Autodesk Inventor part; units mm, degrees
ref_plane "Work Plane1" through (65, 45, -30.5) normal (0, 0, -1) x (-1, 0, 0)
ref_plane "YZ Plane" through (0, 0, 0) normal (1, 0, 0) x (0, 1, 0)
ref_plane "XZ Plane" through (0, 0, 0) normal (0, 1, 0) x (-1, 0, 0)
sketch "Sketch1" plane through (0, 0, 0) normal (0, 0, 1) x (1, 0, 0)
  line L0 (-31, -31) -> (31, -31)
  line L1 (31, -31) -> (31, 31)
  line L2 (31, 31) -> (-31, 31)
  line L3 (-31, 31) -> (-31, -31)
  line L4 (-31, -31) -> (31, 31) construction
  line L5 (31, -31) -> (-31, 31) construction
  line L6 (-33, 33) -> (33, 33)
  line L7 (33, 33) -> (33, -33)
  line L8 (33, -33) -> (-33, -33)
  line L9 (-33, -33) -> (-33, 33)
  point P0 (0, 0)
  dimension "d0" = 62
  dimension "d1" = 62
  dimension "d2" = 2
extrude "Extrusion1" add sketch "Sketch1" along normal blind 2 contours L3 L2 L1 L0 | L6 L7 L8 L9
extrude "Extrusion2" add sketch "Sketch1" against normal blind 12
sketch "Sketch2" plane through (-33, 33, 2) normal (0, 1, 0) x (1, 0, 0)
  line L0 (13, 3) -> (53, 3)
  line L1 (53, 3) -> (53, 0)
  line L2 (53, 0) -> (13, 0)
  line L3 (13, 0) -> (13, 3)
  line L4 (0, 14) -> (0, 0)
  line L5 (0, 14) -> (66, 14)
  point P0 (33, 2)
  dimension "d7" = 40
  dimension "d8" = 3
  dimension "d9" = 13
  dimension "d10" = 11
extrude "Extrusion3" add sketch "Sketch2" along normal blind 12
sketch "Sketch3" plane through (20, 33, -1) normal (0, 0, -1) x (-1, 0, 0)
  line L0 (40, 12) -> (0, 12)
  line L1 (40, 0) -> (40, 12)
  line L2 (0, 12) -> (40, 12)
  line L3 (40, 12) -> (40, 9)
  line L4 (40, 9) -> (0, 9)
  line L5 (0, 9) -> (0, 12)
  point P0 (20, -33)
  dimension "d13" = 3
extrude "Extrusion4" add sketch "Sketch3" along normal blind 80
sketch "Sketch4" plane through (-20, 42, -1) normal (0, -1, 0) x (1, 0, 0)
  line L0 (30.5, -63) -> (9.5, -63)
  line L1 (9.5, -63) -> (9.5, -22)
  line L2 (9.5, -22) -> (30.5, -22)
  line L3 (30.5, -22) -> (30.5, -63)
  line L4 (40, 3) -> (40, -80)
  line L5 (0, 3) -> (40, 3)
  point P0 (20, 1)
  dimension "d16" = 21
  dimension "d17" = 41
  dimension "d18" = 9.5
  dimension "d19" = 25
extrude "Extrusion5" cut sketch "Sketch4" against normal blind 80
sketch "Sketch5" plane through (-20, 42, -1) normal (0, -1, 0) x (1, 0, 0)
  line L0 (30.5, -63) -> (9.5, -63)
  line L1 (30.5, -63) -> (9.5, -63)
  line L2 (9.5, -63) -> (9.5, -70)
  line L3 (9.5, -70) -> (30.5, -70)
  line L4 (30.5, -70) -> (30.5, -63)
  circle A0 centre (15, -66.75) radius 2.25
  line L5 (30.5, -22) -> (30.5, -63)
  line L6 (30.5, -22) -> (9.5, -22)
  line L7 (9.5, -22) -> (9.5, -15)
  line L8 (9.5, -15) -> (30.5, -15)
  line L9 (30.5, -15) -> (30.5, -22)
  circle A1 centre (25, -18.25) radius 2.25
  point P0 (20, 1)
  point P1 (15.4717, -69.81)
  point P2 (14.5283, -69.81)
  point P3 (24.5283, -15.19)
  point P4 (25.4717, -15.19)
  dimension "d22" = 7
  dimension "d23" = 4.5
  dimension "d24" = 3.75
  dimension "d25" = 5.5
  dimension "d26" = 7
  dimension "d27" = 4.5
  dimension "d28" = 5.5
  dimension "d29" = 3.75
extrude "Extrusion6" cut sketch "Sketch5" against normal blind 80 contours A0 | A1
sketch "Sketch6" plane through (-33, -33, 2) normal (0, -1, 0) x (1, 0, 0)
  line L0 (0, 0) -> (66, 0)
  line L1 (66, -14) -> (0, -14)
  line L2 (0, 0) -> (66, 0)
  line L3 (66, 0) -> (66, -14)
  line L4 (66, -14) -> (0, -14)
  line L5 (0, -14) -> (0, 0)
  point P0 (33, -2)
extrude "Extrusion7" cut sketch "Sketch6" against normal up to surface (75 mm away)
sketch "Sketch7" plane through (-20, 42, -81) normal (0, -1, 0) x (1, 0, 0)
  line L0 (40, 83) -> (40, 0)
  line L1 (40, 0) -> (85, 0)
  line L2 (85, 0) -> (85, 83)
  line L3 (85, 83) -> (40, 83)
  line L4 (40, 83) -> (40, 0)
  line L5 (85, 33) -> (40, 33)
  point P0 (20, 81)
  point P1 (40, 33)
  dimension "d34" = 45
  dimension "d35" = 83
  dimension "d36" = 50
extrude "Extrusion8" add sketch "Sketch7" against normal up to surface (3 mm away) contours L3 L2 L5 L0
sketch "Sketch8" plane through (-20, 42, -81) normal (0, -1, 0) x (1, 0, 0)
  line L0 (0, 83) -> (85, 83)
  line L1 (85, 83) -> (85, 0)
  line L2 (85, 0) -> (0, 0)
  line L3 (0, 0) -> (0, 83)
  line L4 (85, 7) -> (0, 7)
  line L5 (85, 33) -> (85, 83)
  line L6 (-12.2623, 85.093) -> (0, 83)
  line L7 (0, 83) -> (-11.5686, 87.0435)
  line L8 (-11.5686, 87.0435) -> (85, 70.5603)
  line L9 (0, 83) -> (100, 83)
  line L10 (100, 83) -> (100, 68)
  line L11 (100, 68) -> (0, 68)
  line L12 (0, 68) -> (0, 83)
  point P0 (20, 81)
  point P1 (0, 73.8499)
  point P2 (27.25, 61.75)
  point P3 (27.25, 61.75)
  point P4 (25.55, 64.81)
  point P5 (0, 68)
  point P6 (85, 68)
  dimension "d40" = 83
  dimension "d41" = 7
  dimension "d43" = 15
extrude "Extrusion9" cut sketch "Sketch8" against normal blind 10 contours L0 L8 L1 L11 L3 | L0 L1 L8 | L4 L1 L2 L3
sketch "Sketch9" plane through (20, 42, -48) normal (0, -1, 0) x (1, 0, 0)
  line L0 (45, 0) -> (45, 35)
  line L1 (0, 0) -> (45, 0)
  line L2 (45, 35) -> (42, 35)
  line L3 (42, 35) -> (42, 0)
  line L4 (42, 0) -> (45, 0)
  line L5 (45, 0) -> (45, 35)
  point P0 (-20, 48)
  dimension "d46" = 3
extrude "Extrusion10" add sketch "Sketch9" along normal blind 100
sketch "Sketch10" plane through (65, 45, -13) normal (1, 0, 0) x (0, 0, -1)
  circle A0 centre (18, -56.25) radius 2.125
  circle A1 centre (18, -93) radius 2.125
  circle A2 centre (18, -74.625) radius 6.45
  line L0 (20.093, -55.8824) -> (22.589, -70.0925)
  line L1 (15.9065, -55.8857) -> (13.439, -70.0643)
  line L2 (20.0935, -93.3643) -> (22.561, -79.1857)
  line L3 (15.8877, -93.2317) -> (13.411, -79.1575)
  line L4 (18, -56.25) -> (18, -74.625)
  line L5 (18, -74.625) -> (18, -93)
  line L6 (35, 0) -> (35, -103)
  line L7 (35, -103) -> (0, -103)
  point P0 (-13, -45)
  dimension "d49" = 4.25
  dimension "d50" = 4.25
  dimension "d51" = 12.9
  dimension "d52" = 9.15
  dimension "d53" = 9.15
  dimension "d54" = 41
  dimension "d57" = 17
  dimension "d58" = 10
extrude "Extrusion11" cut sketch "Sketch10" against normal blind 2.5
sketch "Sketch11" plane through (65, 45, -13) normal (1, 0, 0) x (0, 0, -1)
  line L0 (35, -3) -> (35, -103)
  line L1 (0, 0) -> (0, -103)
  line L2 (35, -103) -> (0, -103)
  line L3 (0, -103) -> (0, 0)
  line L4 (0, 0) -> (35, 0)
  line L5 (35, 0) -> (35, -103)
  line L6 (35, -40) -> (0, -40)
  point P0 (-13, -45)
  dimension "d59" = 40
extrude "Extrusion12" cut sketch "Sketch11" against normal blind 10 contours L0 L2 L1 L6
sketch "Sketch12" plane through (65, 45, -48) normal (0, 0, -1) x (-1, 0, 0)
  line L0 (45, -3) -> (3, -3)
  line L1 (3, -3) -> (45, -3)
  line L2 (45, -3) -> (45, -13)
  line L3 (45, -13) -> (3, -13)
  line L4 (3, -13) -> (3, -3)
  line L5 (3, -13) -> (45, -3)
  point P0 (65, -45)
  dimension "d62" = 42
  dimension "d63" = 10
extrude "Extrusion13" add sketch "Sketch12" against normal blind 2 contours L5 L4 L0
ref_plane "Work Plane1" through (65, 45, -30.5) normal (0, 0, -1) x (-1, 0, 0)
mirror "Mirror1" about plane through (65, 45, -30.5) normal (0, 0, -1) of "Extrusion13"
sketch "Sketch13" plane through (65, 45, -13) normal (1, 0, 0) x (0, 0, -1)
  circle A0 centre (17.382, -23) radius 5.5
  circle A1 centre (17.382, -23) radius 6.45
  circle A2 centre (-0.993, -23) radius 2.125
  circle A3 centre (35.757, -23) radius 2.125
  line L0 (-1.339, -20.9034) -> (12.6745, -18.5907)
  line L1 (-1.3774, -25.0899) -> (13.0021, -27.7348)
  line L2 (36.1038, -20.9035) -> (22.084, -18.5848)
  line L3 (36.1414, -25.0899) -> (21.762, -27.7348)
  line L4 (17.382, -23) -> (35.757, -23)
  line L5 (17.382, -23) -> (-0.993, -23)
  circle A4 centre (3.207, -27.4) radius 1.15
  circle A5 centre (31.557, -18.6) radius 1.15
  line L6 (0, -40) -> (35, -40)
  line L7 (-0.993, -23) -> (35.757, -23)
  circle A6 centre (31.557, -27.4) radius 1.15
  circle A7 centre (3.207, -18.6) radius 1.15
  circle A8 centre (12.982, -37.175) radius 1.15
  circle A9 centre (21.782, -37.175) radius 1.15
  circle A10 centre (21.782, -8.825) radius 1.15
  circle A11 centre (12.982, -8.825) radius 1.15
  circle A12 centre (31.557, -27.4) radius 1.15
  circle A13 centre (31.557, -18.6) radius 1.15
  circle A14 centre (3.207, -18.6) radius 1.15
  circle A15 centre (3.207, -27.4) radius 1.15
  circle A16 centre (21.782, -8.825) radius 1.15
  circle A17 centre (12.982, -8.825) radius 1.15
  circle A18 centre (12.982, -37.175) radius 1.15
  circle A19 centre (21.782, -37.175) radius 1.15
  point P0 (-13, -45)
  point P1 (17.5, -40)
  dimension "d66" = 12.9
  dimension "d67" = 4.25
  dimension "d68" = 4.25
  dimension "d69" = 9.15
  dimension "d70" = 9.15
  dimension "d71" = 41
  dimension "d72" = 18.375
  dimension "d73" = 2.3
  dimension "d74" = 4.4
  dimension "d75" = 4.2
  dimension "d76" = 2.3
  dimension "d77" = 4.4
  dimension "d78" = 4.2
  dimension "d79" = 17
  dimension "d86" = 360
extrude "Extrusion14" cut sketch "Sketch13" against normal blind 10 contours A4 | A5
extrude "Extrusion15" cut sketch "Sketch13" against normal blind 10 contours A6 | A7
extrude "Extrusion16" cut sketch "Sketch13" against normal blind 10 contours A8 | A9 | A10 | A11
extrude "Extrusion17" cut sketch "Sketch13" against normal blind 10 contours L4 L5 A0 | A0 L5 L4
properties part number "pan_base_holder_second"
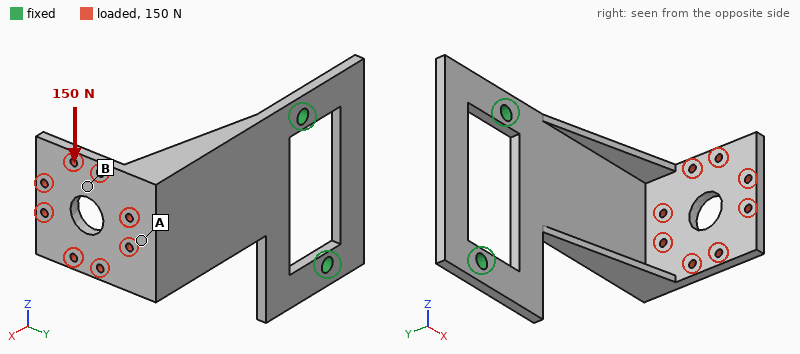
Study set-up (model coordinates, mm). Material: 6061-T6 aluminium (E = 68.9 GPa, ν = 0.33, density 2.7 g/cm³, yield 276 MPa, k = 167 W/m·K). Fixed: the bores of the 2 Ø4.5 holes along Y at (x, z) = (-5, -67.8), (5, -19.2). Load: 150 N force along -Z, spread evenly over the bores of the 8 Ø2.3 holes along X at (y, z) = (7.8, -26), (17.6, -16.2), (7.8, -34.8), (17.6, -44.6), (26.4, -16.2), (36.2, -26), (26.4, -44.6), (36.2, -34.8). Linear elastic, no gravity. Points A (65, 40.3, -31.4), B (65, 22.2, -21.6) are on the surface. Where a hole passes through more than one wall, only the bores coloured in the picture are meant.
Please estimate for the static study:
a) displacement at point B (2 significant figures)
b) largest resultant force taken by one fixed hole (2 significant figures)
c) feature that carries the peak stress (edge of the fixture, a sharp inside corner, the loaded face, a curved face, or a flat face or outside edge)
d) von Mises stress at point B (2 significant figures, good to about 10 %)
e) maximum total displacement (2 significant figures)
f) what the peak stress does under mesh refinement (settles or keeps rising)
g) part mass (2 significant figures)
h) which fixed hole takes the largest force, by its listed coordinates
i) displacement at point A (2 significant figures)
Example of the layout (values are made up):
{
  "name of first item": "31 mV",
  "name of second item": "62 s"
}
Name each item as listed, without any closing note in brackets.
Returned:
{
  "displacement at point B": "0.39 mm",
  "largest resultant force taken by one fixed hole": "210 N",
  "feature that carries the peak stress": "a sharp inside corner",
  "von Mises stress at point B": "8.3 MPa",
  "maximum total displacement": "0.82 mm",
  "what the peak stress does under mesh refinement": "keeps rising",
  "part mass": "37 g",
  "which fixed hole takes the largest force, by its listed coordinates": "(-5, -67.8)",
  "displacement at point A": "0.17 mm"
}
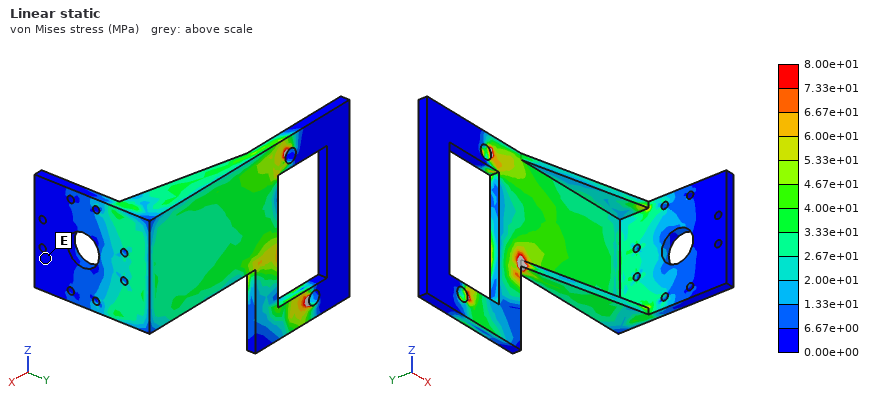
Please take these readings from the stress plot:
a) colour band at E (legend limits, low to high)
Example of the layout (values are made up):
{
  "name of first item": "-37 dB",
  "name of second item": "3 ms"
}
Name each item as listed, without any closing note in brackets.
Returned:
{
  "colour band at E": "0.00e+00 to 6.67e+00 MPa"
}
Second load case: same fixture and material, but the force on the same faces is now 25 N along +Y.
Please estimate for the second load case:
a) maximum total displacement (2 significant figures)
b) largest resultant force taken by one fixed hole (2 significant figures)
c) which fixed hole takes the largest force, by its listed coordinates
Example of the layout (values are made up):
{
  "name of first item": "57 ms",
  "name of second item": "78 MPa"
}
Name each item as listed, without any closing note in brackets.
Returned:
{
  "maximum total displacement": "0.60 mm",
  "largest resultant force taken by one fixed hole": "22 N",
  "which fixed hole takes the largest force, by its listed coordinates": "(5, -19.2)"
}
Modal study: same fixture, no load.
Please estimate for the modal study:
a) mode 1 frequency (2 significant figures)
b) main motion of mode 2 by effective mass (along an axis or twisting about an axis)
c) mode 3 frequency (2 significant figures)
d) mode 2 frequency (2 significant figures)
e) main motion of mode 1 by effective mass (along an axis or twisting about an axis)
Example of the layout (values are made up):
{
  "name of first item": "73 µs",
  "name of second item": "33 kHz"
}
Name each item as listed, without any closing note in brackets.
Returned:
{
  "mode 1 frequency": "280 Hz",
  "main motion of mode 2 by effective mass": "along Z",
  "mode 3 frequency": "1700 Hz",
  "mode 2 frequency": "810 Hz",
  "main motion of mode 1 by effective mass": "along Y"
}
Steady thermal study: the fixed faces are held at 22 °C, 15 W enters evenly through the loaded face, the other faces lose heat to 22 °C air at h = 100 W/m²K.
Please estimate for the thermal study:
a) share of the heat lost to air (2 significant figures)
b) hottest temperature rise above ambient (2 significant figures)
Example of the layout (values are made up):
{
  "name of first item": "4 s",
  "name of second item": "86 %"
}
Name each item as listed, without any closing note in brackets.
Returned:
{
  "share of the heat lost to air": "80 %",
  "hottest temperature rise above ambient": "29 K"
}
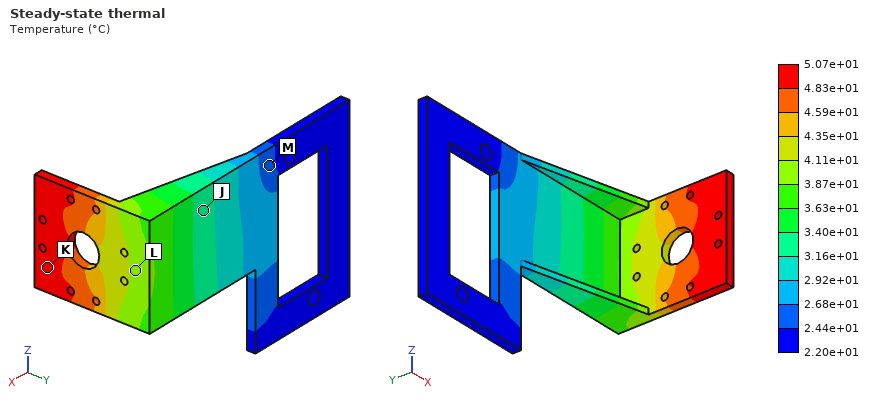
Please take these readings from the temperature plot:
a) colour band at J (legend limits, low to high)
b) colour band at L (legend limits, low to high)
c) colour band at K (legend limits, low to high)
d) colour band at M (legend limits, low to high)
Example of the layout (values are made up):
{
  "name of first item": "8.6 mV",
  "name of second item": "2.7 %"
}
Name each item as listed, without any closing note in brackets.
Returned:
{
  "colour band at J": "3.16e+01 to 3.40e+01 °C",
  "colour band at L": "3.87e+01 to 4.11e+01 °C",
  "colour band at K": "4.83e+01 to 5.07e+01 °C",
  "colour band at M": "2.44e+01 to 2.68e+01 °C"
}
